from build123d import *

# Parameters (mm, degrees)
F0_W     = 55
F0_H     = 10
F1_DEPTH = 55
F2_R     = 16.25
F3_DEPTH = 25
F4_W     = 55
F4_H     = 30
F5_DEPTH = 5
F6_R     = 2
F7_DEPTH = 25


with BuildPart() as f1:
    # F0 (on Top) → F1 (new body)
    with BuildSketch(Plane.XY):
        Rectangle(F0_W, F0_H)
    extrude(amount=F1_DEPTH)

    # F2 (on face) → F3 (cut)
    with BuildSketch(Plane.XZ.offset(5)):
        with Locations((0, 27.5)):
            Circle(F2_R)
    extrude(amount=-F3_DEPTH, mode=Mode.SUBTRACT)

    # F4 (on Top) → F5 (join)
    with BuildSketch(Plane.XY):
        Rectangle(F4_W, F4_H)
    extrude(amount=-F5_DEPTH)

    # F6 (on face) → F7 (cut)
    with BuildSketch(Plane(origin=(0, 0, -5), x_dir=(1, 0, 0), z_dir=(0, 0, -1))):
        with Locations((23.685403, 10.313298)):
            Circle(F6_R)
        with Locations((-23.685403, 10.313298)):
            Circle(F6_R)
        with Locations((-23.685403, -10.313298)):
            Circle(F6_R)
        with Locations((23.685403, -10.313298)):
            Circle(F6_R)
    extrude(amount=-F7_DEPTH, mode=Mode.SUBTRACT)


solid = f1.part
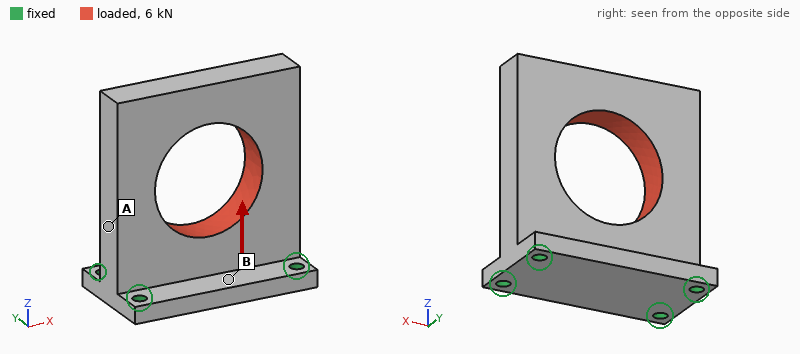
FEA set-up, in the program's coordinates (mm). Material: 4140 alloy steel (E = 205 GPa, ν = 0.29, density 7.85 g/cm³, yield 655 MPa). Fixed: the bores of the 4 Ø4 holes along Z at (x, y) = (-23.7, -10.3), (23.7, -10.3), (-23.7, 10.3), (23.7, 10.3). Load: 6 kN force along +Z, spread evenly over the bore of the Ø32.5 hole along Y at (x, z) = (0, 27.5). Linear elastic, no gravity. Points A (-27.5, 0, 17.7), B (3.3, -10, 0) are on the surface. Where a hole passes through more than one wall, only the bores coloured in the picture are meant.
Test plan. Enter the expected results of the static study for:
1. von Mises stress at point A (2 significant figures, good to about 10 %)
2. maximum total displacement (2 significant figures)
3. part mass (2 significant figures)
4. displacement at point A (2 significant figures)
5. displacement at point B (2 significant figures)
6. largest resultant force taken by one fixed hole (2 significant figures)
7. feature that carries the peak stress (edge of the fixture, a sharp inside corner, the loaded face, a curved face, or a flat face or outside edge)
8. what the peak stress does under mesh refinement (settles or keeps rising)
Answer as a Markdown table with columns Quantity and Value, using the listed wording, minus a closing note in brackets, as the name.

| Quantity | Value |
|---|---|
| von Mises stress at point A | 19 MPa |
| maximum total displacement | 9.4 µm |
| part mass | 240 g |
| displacement at point A | 5.5 µm |
| displacement at point B | 4.8 µm |
| largest resultant force taken by one fixed hole | 1.6 kN |
| feature that carries the peak stress | edge of the fixture |
| what the peak stress does under mesh refinement | keeps rising |
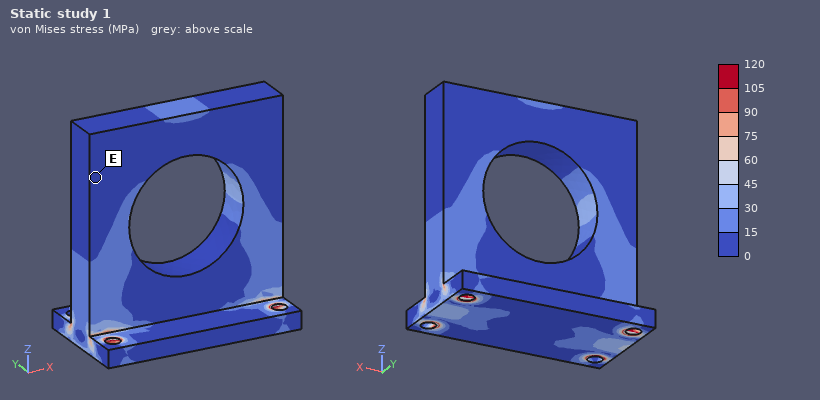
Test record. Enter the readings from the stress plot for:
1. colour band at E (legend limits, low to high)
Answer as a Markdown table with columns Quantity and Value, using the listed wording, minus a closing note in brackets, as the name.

| Quantity | Value |
|---|---|
| colour band at E | 0 to 15 MPa |
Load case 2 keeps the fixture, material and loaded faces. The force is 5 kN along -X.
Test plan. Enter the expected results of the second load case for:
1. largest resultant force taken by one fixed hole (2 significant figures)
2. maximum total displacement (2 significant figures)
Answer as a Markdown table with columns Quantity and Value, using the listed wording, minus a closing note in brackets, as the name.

| Quantity | Value |
|---|---|
| largest resultant force taken by one fixed hole | 2.1 kN |
| maximum total displacement | 35 µm |
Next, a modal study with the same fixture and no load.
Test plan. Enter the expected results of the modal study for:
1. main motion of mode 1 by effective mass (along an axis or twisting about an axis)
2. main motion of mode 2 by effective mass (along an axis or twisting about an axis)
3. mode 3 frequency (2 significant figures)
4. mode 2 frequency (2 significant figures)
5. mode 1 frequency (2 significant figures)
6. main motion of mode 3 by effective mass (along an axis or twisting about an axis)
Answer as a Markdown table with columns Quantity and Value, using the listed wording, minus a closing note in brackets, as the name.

| Quantity | Value |
|---|---|
| main motion of mode 1 by effective mass | along Y |
| main motion of mode 2 by effective mass | twisting about Z |
| mode 3 frequency | 5100 Hz |
| mode 2 frequency | 4500 Hz |
| mode 1 frequency | 1900 Hz |
| main motion of mode 3 by effective mass | along X |
